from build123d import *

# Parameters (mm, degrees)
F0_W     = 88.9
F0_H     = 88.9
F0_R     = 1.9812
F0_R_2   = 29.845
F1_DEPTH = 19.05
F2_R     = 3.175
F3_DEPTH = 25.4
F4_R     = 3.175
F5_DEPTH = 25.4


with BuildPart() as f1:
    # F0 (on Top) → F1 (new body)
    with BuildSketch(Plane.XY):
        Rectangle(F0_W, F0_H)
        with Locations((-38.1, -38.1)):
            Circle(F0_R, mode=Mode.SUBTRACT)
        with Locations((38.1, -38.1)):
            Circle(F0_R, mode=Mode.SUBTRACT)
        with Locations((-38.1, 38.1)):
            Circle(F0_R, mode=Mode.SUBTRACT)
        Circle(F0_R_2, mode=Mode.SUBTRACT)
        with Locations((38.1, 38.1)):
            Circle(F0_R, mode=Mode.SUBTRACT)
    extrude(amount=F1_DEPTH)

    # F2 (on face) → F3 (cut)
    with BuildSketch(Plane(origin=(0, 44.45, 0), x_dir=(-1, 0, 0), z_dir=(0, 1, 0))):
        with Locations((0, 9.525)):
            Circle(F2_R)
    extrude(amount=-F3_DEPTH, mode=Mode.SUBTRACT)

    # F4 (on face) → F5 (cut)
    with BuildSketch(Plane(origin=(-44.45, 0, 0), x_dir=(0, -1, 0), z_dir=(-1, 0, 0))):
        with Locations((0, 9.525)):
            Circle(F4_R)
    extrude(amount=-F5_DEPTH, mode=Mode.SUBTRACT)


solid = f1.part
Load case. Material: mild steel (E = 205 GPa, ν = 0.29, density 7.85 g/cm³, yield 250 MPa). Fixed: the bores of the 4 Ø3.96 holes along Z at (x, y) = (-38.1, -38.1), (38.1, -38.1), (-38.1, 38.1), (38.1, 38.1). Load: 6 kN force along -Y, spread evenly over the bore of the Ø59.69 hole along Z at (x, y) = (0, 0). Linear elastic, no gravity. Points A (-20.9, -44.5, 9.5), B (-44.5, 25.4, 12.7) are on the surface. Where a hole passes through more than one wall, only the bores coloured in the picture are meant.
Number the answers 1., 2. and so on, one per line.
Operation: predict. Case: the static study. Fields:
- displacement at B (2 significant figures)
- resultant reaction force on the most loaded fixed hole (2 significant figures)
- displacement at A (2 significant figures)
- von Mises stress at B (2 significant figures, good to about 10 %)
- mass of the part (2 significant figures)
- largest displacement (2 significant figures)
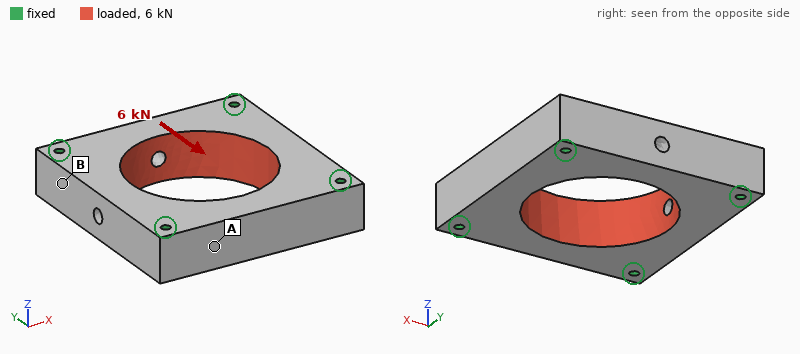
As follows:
1. 0.35 µm
2. 1.6 kN
3. 1.2 µm
4. 6.1 MPa
5. 750 g
6. 2.2 µm
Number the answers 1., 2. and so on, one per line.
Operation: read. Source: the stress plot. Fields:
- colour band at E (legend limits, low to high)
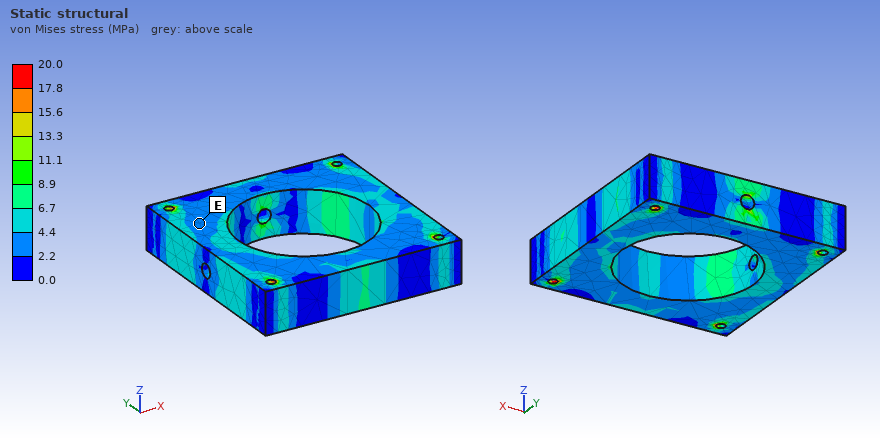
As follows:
1. 2.2 to 4.4 MPa
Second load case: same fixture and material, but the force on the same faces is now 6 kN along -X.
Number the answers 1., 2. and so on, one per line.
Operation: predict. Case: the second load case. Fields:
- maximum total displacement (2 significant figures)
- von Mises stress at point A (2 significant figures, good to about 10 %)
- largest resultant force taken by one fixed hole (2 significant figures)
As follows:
1. 2.2 µm
2. 6.7 MPa
3. 1.6 kN
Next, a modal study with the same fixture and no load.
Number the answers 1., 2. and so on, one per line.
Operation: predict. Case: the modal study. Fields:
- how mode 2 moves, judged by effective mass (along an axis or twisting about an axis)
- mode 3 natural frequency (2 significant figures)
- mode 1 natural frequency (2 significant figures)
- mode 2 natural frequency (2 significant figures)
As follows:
1. along Z
2. 12 kHz
3. 7600 Hz
4. 11 kHz
